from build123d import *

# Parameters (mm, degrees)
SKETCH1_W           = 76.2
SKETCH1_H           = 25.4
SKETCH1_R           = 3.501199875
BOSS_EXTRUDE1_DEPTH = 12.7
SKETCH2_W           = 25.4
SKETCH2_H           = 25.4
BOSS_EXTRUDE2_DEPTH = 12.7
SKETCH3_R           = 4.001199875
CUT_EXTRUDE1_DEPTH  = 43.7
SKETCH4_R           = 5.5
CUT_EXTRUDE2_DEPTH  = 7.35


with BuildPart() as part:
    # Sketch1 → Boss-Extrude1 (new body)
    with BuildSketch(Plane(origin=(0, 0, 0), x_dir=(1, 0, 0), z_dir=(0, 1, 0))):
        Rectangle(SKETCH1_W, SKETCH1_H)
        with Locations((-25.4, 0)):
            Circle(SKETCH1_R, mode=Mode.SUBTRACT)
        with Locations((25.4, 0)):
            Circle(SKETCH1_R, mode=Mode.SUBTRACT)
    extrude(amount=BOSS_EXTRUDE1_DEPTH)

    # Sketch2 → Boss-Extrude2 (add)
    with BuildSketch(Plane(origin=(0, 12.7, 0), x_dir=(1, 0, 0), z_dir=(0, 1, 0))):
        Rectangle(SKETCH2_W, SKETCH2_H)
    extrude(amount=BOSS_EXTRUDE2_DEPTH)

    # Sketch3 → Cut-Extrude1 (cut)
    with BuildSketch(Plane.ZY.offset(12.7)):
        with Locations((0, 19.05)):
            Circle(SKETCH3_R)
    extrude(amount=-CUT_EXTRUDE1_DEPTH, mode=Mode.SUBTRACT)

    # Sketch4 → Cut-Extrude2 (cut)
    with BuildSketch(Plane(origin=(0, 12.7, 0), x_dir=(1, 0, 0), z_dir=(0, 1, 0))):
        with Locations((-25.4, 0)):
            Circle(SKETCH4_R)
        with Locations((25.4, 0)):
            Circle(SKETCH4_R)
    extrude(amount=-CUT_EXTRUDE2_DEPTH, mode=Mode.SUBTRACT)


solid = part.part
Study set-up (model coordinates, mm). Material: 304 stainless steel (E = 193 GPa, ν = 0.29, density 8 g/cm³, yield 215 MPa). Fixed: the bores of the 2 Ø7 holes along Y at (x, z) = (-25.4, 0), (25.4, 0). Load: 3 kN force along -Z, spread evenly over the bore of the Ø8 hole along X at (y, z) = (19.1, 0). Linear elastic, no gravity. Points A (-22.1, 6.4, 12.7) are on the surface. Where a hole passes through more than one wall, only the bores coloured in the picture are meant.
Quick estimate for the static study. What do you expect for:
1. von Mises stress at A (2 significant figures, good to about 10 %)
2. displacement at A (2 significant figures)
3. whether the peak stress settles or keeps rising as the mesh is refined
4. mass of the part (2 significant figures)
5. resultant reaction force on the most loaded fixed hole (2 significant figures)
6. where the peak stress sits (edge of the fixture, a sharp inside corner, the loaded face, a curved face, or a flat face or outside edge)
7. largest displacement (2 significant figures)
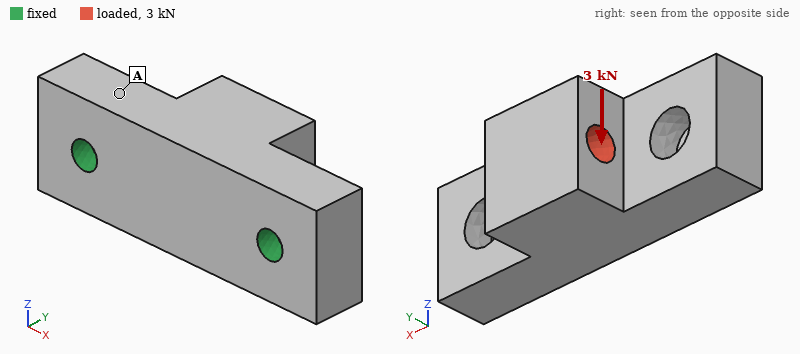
26 MPa
8.7 µm
keeps rising
240 g
1.5 kN
edge of the fixture
26 µm
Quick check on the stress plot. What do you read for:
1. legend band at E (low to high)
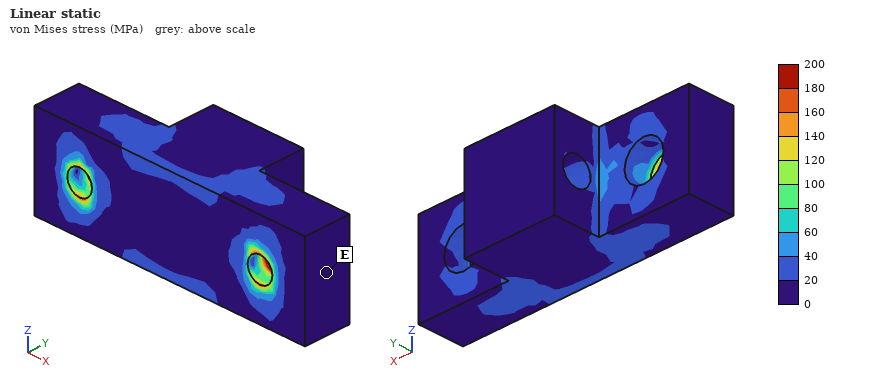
0 to 20 MPa
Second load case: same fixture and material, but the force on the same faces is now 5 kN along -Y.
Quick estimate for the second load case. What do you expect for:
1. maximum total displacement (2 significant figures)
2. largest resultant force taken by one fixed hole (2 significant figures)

6.7 µm
3.1 kN
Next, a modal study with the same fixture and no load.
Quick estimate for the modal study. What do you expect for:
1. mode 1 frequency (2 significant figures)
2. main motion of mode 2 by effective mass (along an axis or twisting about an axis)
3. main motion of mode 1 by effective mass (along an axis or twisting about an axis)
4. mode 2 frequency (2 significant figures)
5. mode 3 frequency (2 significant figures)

6600 Hz
along Y
along Z
13 kHz
18 kHz
